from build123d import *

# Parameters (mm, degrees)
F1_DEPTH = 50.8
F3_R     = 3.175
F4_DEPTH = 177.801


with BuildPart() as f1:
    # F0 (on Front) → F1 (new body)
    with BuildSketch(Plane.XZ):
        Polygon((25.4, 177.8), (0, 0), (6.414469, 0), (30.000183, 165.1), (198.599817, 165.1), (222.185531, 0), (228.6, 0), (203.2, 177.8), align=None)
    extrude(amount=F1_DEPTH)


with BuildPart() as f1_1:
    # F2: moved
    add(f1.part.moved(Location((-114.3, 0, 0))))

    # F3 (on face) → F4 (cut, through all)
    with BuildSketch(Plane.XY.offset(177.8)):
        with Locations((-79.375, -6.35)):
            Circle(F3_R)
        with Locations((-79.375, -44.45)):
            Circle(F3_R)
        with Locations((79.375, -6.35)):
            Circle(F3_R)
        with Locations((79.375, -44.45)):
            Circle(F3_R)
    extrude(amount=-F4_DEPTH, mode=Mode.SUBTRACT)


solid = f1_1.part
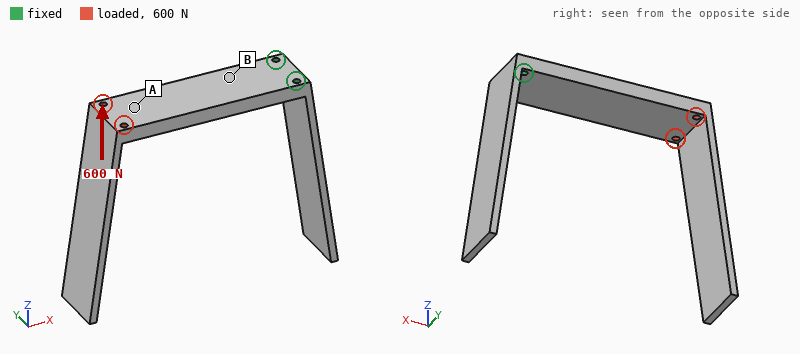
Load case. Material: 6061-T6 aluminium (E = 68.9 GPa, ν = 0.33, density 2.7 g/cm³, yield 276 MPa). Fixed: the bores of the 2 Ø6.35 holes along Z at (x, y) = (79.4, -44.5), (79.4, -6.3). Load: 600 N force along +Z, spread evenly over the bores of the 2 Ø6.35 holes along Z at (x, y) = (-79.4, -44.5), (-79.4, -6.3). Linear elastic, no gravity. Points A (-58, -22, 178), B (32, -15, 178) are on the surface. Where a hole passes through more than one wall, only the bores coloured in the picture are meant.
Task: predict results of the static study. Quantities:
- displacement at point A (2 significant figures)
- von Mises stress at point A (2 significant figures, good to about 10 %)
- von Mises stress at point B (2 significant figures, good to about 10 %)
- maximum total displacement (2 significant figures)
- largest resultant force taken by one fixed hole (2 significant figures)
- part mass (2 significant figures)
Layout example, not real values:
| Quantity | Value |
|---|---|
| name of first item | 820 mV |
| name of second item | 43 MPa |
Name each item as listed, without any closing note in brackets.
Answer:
| Quantity | Value |
|---|---|
| displacement at point A | 1.1 mm |
| von Mises stress at point A | 9.3 MPa |
| von Mises stress at point B | 49 MPa |
| maximum total displacement | 2.9 mm |
| largest resultant force taken by one fixed hole | 300 N |
| part mass | 600 g |
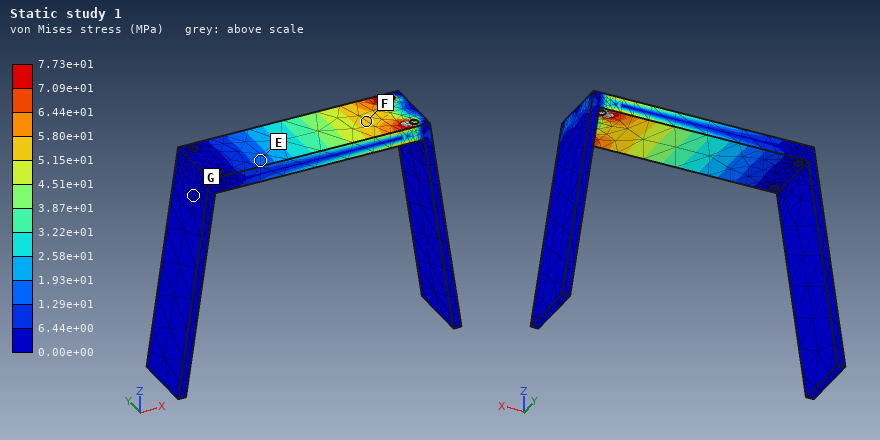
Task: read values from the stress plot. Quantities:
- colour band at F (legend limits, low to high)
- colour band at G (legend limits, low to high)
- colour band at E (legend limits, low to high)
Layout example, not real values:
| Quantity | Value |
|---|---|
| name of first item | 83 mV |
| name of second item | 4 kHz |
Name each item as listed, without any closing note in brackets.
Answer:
| Quantity | Value |
|---|---|
| colour band at F | 5.15e+01 to 5.80e+01 MPa |
| colour band at G | 0.00e+00 to 6.44e+00 MPa |
| colour band at E | 1.29e+01 to 1.93e+01 MPa |
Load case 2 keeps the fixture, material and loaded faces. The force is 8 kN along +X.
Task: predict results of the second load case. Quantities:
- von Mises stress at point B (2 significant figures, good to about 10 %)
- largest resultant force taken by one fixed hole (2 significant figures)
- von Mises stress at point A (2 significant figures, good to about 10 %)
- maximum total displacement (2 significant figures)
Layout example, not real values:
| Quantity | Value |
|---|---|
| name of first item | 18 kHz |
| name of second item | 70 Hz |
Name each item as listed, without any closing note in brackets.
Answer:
| Quantity | Value |
|---|---|
| von Mises stress at point B | 12 MPa |
| largest resultant force taken by one fixed hole | 4.0 kN |
| von Mises stress at point A | 9.6 MPa |
| maximum total displacement | 34 µm |
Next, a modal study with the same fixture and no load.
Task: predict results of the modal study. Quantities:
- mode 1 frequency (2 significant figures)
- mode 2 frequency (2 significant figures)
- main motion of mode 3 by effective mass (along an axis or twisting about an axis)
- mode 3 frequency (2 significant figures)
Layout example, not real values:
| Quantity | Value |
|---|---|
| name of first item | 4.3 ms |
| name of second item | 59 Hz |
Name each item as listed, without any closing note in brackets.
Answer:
| Quantity | Value |
|---|---|
| mode 1 frequency | 130 Hz |
| mode 2 frequency | 180 Hz |
| main motion of mode 3 by effective mass | along Y |
| mode 3 frequency | 270 Hz |
